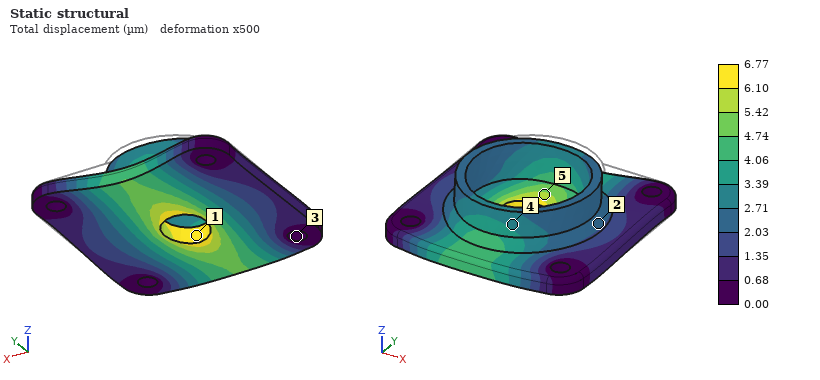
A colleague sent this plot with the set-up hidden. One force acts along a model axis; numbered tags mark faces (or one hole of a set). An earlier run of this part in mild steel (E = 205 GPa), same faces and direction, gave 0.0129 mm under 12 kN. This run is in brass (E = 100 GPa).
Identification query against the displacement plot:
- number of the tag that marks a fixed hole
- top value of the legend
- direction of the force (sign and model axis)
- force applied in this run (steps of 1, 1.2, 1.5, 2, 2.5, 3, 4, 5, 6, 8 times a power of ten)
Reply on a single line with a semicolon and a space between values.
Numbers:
3; 6.77 µm; -Y; 3 kN
